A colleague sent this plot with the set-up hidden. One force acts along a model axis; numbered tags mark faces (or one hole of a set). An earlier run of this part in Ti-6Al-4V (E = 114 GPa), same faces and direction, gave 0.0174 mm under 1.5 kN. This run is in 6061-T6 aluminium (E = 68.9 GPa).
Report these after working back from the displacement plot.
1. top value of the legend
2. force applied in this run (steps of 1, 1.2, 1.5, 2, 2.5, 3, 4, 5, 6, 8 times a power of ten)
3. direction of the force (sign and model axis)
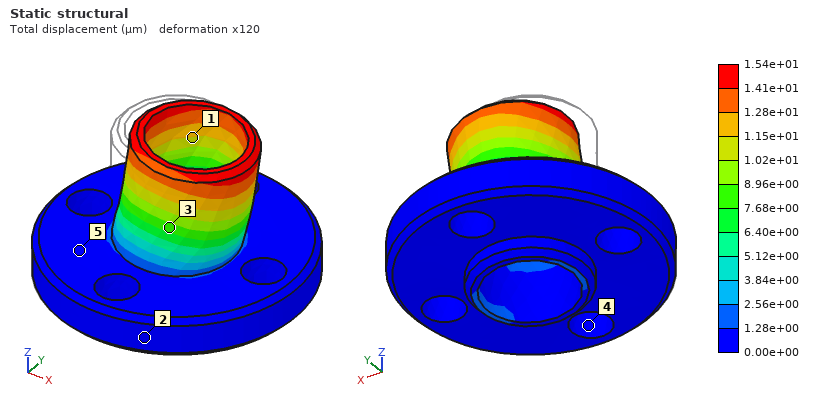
1.54e+01 µm
800 N
+X
